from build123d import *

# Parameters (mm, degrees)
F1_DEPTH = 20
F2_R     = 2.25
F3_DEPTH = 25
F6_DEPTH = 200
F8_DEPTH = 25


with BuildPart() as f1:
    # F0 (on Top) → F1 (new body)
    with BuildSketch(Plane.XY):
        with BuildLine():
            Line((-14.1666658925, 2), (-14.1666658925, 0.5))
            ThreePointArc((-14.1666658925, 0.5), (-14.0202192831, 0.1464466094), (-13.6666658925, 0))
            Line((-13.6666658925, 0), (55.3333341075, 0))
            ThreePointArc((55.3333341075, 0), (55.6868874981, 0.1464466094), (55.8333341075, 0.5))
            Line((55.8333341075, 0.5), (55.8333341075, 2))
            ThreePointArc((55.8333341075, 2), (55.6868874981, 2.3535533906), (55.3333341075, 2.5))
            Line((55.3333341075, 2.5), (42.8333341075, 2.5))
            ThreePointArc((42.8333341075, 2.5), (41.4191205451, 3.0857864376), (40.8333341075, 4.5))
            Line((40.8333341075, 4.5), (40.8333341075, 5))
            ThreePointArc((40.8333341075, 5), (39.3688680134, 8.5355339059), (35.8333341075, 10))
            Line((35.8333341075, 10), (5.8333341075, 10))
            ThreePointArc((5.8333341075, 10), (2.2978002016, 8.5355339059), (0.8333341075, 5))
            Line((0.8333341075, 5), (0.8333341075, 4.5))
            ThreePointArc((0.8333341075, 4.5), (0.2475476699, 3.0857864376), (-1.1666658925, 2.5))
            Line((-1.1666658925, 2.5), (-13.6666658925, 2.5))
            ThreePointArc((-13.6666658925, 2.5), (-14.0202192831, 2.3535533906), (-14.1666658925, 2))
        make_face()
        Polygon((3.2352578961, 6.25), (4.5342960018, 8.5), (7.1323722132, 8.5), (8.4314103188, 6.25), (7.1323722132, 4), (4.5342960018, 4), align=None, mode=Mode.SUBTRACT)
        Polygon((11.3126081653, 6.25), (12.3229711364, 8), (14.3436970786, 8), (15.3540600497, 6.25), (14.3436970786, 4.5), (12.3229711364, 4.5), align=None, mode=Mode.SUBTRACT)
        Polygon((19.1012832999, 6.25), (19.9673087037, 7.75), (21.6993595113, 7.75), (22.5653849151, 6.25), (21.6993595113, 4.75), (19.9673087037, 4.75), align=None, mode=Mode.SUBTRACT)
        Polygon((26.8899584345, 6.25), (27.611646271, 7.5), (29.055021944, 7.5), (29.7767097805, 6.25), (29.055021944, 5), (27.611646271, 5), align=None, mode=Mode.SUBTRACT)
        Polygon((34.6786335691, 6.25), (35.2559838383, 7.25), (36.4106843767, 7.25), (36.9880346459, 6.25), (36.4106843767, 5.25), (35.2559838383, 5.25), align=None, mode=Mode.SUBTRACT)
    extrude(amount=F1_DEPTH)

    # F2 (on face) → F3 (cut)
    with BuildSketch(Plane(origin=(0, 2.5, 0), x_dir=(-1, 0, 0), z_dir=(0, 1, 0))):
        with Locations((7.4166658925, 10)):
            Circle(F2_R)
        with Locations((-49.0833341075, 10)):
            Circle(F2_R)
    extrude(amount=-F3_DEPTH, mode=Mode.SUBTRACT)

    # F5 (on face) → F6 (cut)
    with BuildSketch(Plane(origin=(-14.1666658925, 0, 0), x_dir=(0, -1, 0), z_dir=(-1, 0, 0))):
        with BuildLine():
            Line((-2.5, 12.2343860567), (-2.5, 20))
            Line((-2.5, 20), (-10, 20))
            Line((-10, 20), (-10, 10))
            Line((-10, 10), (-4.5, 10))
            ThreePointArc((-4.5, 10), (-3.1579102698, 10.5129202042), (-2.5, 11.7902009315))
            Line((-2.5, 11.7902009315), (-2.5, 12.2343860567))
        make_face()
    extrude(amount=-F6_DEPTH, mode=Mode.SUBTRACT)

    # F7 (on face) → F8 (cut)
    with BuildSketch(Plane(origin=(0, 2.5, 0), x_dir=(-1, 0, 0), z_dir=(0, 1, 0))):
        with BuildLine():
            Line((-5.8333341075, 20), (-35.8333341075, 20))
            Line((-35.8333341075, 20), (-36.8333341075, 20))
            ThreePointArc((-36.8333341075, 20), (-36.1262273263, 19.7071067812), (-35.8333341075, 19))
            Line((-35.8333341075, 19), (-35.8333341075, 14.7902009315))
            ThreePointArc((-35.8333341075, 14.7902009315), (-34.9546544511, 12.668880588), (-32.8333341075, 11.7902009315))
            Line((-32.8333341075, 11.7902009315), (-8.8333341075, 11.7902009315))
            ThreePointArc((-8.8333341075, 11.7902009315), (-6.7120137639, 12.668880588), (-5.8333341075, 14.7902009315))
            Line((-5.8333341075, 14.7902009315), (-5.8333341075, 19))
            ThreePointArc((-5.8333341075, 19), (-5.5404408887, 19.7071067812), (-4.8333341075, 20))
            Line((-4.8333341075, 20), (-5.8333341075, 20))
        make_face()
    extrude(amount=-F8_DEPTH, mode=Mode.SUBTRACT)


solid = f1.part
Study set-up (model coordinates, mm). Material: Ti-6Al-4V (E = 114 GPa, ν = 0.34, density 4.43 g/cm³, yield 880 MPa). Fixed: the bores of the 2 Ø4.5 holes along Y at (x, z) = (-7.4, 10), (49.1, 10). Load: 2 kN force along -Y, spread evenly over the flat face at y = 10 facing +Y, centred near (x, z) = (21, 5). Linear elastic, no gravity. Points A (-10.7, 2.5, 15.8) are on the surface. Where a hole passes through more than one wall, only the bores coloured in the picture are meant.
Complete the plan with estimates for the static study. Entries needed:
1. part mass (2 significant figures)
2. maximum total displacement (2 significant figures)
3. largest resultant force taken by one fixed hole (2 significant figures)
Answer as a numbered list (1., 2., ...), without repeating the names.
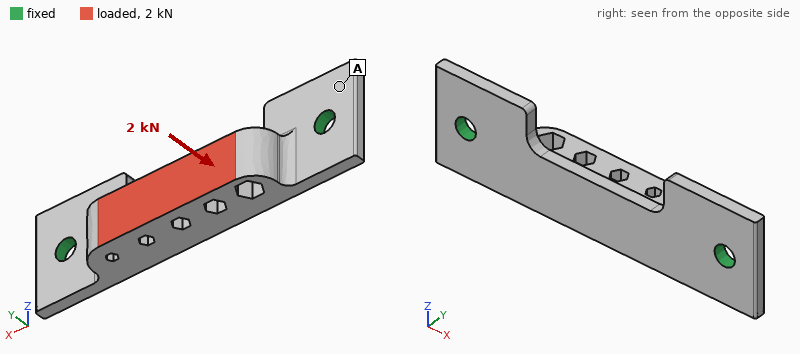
1. 24 g
2. 0.14 mm
3. 1.4 kN
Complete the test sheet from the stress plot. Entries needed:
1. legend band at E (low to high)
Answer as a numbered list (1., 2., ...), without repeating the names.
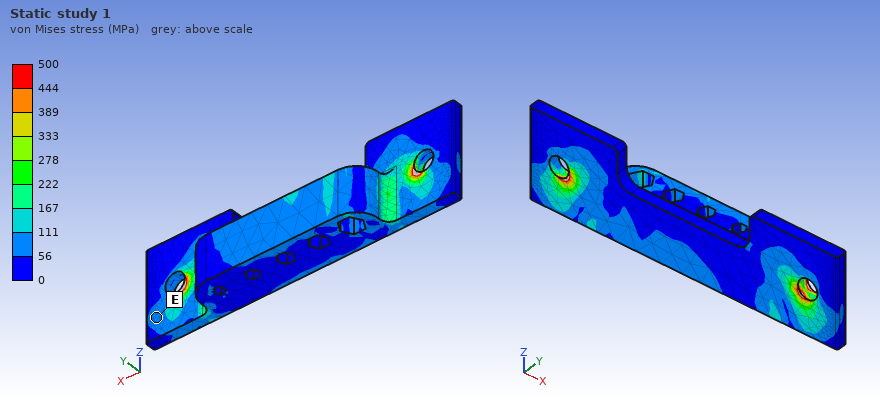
1. 56 to 111 MPa
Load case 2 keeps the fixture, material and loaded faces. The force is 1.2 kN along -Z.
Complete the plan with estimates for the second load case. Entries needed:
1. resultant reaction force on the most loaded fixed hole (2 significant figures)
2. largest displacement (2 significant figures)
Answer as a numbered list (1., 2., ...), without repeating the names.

1. 730 N
2. 0.14 mm
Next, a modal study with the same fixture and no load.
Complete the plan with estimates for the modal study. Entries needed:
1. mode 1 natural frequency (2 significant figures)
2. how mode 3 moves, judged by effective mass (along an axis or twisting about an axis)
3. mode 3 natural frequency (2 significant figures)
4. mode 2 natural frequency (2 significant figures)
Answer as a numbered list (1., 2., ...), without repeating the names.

1. 5400 Hz
2. along Z
3. 13 kHz
4. 9300 Hz
